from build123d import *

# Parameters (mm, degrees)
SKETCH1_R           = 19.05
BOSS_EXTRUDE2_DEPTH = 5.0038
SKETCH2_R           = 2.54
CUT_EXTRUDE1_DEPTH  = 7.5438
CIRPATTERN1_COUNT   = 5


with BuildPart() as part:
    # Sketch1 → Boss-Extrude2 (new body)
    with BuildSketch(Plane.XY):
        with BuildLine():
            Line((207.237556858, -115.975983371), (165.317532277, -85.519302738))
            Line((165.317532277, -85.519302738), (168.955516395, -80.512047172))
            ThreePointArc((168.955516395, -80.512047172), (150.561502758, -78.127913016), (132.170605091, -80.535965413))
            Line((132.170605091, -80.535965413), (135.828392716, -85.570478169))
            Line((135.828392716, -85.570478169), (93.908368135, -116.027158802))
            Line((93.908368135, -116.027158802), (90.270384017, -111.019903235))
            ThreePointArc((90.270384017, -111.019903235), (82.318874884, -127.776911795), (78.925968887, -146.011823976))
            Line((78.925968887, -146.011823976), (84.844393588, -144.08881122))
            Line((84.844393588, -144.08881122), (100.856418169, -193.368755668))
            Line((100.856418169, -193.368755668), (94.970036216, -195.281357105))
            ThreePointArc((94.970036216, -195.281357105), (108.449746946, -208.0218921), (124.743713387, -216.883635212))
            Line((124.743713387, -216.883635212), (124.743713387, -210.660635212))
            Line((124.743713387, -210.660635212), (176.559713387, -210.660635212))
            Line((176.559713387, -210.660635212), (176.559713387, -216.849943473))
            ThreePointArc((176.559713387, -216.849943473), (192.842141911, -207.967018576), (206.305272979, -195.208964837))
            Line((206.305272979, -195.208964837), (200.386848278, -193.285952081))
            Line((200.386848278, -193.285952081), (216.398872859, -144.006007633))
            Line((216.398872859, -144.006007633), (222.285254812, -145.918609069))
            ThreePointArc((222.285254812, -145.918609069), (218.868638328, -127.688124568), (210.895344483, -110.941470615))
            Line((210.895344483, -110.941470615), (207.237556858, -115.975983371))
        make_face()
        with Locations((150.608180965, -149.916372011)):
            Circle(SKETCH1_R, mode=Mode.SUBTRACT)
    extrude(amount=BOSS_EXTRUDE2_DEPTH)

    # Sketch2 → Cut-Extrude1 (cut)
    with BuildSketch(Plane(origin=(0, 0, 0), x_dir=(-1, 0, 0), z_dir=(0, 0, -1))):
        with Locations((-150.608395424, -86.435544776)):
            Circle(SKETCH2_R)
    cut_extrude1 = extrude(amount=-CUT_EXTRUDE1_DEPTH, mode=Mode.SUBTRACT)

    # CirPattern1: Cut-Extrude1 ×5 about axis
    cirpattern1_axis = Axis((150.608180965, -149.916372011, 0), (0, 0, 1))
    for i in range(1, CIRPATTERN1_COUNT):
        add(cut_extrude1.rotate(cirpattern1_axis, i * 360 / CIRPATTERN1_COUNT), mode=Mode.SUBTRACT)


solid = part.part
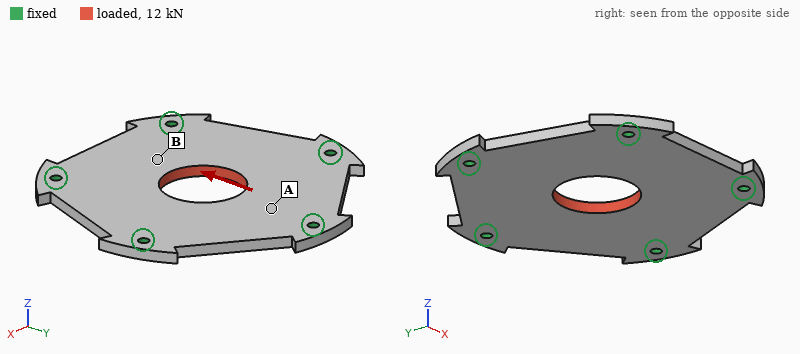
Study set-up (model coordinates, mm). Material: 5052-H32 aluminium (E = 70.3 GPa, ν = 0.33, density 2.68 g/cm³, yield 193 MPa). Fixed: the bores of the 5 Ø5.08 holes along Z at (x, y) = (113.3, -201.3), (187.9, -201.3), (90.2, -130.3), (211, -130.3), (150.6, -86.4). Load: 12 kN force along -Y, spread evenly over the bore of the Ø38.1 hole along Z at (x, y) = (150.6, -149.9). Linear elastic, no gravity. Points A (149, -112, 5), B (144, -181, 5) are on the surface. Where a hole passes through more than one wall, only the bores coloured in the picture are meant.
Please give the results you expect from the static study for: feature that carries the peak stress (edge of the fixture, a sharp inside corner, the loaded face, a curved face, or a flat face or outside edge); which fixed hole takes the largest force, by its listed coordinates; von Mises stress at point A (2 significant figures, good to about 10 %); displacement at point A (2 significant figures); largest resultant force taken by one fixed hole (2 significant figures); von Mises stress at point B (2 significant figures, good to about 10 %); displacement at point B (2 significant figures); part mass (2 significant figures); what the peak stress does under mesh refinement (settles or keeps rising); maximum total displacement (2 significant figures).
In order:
edge of the fixture
(150.6, -86.4)
27 MPa
12 µm
3.6 kN
14 MPa
16 µm
170 g
keeps rising
19 µm
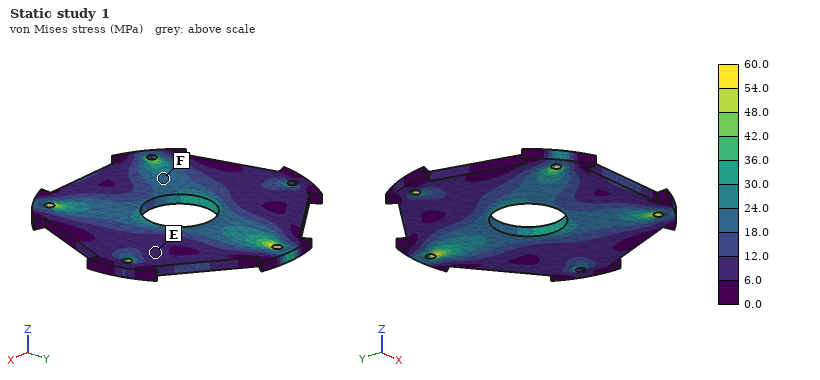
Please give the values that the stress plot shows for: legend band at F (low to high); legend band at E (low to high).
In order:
18.0 to 24.0 MPa
6.0 to 12.0 MPa
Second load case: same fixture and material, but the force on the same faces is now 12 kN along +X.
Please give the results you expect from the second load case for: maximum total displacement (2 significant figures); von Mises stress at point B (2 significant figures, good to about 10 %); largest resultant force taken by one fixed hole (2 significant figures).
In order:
19 µm
17 MPa
3.4 kN
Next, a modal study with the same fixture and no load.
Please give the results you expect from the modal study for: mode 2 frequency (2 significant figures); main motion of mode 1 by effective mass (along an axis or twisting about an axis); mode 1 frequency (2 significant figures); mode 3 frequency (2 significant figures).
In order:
4200 Hz
along Z
2500 Hz
4200 Hz
